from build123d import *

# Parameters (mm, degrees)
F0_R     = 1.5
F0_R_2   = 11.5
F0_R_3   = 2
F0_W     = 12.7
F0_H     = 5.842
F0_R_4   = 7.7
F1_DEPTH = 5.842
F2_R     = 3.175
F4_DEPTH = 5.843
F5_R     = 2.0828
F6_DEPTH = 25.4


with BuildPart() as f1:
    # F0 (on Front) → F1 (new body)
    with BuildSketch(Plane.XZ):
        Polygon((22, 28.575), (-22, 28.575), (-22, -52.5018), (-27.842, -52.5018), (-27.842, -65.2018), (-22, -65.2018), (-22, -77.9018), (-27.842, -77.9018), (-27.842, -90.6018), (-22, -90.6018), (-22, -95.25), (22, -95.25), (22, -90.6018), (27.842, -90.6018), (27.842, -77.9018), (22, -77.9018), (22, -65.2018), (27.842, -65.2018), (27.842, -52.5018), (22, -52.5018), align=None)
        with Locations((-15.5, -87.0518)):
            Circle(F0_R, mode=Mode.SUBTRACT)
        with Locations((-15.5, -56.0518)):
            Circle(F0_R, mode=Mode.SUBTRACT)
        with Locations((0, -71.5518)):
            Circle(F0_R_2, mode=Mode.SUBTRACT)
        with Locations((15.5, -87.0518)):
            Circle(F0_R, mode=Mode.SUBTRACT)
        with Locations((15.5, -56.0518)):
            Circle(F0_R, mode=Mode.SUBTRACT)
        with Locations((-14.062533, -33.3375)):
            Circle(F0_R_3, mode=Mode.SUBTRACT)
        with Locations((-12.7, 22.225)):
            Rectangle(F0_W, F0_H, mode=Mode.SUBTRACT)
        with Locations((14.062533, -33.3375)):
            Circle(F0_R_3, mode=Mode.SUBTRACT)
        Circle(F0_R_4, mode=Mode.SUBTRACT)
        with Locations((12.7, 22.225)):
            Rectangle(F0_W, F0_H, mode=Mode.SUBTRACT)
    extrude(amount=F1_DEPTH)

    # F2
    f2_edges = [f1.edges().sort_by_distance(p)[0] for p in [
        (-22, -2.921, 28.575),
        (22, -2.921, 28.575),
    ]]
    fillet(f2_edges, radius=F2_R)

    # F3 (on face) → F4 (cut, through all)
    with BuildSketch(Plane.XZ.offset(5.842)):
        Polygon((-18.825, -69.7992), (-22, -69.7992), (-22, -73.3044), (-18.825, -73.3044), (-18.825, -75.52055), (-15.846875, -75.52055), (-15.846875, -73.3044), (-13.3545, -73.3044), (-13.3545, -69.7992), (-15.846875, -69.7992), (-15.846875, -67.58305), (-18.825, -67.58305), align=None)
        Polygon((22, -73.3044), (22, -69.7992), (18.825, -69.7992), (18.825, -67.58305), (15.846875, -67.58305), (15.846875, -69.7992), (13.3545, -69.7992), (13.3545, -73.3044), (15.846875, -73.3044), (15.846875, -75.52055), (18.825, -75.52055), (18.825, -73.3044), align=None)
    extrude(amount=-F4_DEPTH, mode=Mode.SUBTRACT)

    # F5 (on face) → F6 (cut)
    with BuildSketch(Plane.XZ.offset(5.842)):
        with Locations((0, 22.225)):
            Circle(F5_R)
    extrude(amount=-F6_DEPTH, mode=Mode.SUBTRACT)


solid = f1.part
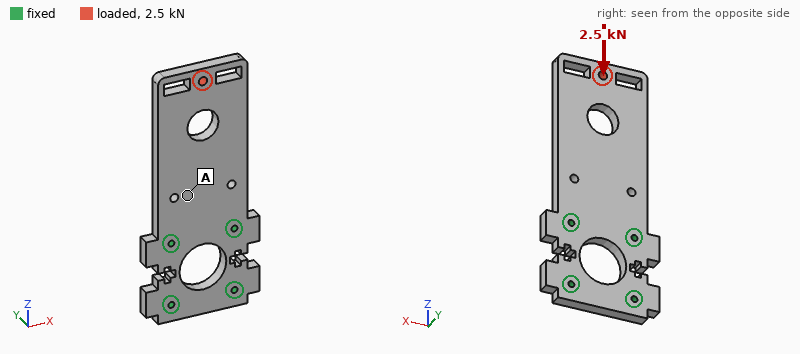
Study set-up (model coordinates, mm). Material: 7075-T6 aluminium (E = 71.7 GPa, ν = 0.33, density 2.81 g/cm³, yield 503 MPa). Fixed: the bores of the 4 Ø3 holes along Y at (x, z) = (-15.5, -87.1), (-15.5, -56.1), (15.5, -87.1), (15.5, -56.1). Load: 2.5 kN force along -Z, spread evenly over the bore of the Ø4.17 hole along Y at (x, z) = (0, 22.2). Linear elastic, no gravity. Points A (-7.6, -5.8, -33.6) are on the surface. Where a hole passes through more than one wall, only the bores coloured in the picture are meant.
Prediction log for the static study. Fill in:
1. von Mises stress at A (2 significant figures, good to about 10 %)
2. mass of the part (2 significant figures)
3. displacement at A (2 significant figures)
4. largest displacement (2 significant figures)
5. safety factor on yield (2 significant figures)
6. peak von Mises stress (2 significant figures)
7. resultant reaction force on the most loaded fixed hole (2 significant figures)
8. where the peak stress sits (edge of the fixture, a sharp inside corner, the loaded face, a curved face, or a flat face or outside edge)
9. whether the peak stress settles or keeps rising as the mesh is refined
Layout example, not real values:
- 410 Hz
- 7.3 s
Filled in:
- 8.4 MPa
- 79 g
- 4.2 µm
- 24 µm
- 6.6
- 77 MPa
- 1.2 kN
- the loaded face
- settles
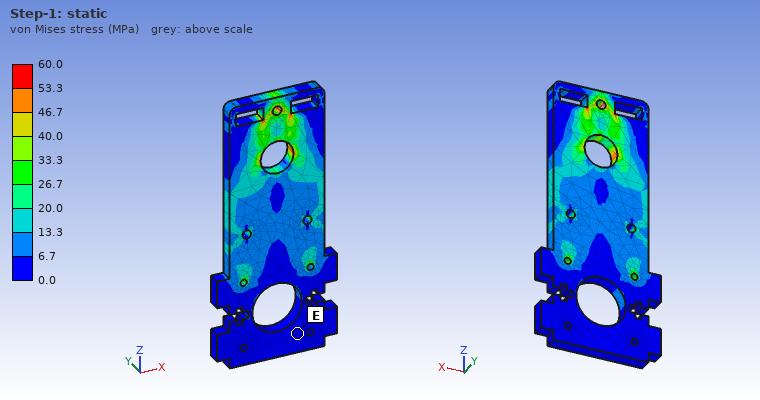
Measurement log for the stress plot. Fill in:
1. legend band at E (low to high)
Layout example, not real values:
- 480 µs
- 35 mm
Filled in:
- 0.0 to 6.7 MPa
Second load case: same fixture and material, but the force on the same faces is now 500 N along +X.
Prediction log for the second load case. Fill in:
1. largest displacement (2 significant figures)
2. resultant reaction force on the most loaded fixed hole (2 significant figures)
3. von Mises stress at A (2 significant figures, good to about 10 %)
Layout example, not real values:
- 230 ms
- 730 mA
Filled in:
- 47 µm
- 1.2 kN
- 7.3 MPa
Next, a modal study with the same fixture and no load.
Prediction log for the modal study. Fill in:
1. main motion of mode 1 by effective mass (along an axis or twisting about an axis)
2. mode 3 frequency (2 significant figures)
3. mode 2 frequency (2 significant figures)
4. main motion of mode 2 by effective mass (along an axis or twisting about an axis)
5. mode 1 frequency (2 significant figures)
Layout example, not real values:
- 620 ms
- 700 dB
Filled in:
- along Y
- 3900 Hz
- 2700 Hz
- twisting about Z
- 690 Hz
